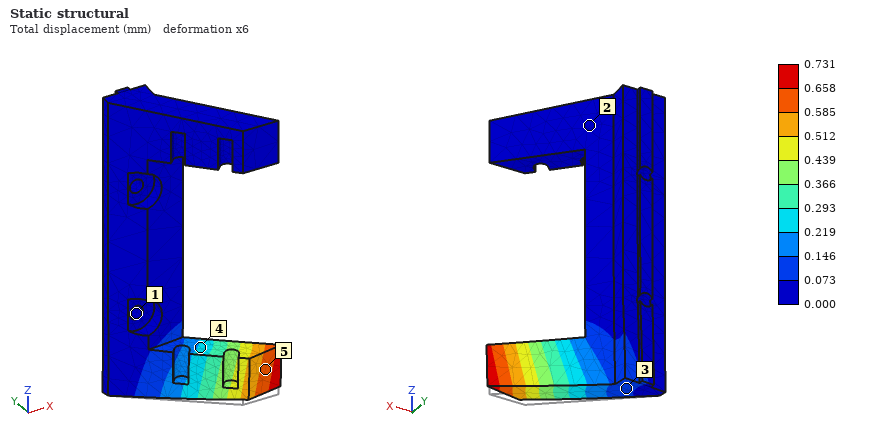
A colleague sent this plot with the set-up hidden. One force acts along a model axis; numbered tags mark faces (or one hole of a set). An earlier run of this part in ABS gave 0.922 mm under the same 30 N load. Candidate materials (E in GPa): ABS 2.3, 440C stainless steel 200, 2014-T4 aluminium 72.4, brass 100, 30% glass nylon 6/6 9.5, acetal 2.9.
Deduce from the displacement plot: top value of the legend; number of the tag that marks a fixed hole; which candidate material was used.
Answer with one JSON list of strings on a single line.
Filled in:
["0.731 mm", "1", "acetal"]
